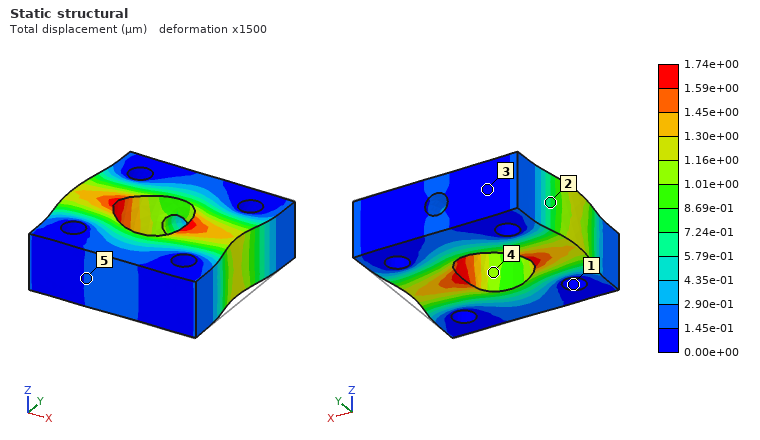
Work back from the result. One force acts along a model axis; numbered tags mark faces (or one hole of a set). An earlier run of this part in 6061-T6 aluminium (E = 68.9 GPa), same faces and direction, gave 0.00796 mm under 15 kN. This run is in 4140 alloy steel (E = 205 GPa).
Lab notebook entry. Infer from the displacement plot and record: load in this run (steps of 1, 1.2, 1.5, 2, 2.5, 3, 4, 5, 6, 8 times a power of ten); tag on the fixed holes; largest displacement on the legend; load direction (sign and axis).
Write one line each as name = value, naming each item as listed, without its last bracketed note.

load in this run = 10 kN
tag on the fixed holes = 1
largest displacement on the legend = 1.74e+00 µm
load direction = -X
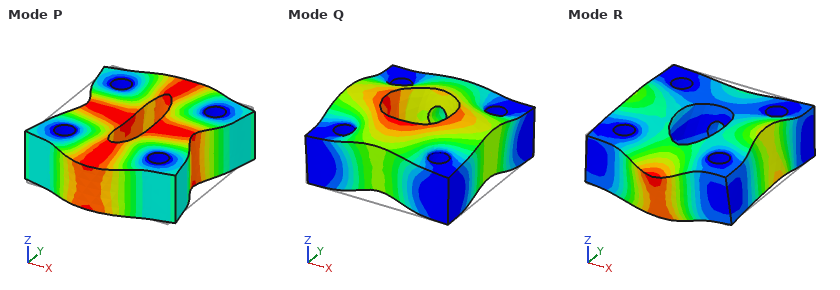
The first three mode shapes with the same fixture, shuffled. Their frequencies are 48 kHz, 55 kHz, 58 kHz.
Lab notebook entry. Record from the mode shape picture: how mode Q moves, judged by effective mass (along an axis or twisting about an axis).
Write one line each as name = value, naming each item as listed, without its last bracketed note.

how mode Q moves, judged by effective mass = along Z
